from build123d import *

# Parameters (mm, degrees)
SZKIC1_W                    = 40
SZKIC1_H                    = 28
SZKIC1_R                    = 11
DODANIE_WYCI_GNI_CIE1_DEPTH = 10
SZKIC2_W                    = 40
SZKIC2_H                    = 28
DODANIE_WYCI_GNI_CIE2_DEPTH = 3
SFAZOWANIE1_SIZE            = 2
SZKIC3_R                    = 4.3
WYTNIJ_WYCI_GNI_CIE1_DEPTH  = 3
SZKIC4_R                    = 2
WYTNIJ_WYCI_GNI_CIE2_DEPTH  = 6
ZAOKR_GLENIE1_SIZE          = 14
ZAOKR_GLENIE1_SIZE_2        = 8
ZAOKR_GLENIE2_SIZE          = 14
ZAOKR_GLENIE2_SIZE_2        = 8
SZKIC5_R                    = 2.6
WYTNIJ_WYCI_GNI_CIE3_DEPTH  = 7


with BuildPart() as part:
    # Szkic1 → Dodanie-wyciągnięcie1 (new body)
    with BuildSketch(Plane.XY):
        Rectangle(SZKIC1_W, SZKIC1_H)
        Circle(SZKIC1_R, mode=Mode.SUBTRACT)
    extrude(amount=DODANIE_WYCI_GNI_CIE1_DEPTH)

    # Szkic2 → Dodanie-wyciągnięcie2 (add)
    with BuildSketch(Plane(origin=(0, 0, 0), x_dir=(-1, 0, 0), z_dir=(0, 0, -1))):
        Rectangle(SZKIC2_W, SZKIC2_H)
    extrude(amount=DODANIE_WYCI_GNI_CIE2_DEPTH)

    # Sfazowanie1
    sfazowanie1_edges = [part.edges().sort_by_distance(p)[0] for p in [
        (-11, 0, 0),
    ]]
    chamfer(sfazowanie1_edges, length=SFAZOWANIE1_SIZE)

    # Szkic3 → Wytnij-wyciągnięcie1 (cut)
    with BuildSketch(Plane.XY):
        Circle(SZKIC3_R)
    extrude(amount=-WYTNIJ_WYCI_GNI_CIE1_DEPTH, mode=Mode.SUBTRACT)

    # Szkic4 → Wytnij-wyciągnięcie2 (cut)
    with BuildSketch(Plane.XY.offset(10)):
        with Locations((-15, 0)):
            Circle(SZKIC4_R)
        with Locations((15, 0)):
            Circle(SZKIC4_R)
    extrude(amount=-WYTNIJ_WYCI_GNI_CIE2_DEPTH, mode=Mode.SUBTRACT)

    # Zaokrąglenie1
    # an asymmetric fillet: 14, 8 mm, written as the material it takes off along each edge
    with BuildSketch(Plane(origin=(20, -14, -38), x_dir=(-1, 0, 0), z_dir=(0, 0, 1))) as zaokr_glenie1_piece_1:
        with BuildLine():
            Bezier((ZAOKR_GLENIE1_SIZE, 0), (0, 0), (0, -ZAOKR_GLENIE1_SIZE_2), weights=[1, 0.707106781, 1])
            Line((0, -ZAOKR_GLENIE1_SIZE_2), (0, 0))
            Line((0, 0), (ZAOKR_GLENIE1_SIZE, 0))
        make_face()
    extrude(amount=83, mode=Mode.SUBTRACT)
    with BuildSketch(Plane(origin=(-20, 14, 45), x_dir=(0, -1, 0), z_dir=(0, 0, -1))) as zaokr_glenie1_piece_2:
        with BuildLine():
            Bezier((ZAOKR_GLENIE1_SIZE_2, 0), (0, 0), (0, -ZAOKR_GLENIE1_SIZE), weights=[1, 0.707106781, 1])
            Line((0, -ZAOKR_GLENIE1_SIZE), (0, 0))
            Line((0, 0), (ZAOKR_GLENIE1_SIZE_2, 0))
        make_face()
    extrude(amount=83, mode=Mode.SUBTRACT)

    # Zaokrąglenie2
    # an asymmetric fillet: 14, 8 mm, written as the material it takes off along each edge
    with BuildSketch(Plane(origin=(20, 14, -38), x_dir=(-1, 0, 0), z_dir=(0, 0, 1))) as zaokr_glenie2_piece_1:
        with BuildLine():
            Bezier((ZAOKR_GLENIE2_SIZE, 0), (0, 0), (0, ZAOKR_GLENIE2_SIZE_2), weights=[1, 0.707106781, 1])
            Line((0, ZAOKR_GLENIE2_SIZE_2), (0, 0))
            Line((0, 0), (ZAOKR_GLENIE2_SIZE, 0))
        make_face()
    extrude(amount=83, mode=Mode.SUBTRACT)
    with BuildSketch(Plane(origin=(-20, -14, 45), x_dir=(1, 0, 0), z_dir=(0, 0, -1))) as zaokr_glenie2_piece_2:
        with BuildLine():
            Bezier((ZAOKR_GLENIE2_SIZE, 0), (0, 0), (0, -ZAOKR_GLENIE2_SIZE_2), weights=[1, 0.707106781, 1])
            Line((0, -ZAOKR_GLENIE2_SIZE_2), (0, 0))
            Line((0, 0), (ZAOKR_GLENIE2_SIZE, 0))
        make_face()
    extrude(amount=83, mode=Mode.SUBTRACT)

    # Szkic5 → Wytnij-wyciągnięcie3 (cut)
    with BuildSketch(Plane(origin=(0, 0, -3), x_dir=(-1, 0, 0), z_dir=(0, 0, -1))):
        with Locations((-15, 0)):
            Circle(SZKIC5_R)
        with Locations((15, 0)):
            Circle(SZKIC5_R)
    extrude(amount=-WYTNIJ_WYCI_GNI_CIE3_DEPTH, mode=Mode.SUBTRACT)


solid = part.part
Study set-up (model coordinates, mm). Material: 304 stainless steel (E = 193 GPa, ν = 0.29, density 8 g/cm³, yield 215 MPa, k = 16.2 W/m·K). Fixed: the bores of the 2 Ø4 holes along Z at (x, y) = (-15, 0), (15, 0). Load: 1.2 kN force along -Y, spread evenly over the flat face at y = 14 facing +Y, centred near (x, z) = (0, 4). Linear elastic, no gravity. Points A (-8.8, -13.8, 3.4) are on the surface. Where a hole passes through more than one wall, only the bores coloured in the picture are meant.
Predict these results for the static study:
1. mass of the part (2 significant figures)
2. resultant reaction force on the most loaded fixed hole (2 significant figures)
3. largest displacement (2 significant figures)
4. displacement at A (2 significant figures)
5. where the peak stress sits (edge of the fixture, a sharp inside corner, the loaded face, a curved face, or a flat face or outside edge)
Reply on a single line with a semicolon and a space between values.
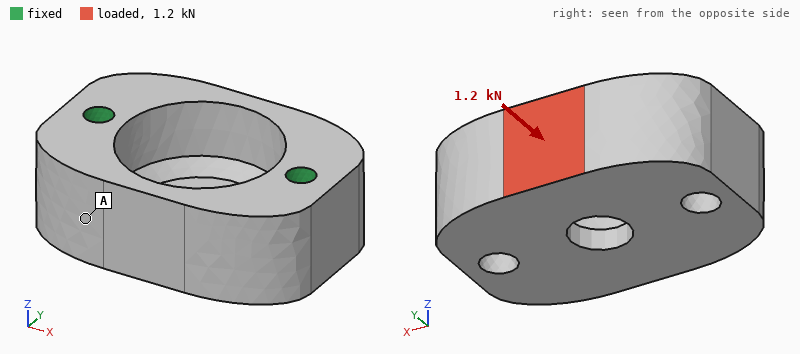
72 g; 670 N; 3.4 µm; 1.2 µm; edge of the fixture
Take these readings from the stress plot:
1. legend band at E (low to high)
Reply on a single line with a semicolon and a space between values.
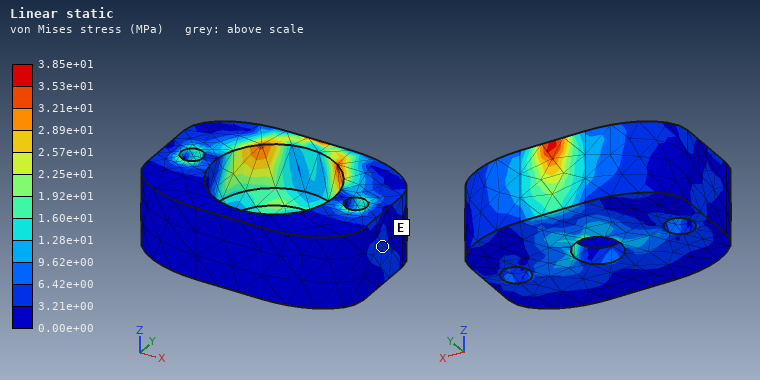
3.21e+00 to 6.42e+00 MPa
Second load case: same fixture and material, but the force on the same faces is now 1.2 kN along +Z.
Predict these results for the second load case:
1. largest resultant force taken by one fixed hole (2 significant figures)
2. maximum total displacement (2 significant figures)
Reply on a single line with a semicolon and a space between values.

730 N; 10 µm
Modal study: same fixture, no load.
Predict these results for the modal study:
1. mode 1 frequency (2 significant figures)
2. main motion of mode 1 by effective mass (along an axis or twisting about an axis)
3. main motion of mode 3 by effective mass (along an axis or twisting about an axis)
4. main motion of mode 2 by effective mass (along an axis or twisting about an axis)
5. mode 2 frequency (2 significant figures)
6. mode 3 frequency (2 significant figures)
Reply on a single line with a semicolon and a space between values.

13 kHz; along Y; along Z; twisting about Z; 22 kHz; 24 kHz
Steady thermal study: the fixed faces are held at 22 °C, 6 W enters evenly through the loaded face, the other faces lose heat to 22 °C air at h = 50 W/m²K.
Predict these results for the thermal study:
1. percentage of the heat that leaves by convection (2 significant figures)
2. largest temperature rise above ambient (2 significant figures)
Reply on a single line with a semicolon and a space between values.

27 %; 37 K
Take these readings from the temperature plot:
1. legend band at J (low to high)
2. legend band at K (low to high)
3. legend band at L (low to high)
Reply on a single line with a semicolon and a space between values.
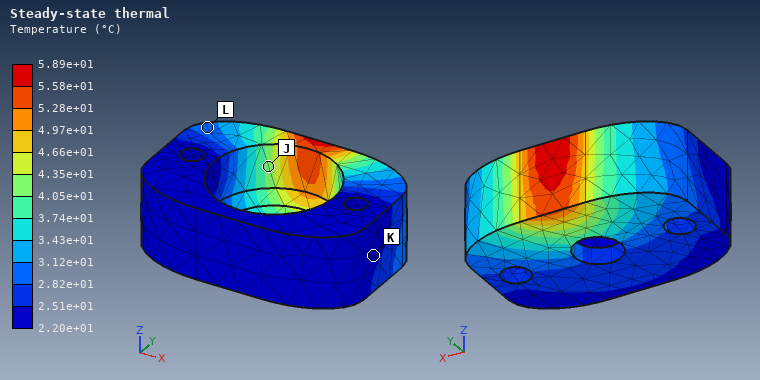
4.05e+01 to 4.35e+01 °C; 2.20e+01 to 2.51e+01 °C; 2.82e+01 to 3.12e+01 °C
